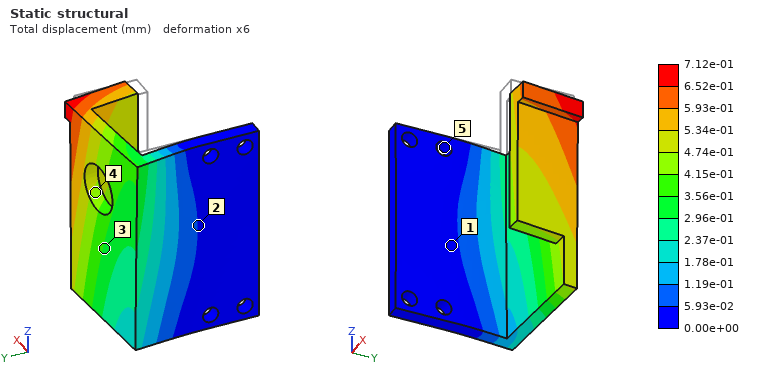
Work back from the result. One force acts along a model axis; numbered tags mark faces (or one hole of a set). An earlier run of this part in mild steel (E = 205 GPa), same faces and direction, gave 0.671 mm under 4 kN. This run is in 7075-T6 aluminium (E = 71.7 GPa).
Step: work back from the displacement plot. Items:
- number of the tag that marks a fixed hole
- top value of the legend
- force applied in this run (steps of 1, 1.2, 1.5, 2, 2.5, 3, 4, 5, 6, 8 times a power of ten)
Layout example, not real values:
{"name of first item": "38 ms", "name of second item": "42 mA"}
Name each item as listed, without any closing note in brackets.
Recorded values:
{"number of the tag that marks a fixed hole": "5", "top value of the legend": "7.12e-01 mm", "force applied in this run": "1.5 kN"}
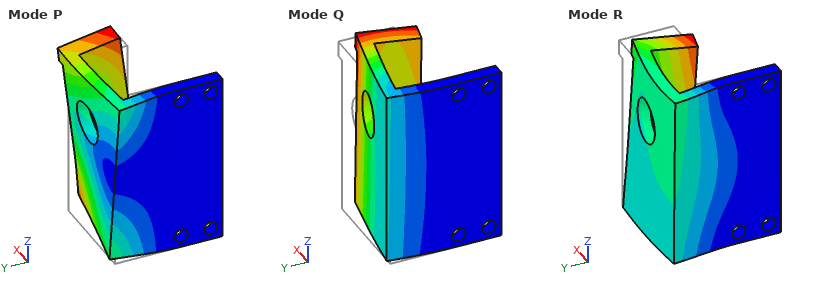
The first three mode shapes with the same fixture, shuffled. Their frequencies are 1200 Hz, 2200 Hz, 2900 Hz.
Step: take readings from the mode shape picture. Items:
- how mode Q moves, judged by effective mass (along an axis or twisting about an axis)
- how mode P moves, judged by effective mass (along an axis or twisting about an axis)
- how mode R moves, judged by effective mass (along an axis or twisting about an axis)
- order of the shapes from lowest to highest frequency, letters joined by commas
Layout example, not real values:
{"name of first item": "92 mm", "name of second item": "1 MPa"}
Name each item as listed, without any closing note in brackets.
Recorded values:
{"how mode Q moves, judged by effective mass": "along Y", "how mode P moves, judged by effective mass": "along Z", "how mode R moves, judged by effective mass": "along X", "order of the shapes from lowest to highest frequency, letters joined by commas": "Q, P, R"}
